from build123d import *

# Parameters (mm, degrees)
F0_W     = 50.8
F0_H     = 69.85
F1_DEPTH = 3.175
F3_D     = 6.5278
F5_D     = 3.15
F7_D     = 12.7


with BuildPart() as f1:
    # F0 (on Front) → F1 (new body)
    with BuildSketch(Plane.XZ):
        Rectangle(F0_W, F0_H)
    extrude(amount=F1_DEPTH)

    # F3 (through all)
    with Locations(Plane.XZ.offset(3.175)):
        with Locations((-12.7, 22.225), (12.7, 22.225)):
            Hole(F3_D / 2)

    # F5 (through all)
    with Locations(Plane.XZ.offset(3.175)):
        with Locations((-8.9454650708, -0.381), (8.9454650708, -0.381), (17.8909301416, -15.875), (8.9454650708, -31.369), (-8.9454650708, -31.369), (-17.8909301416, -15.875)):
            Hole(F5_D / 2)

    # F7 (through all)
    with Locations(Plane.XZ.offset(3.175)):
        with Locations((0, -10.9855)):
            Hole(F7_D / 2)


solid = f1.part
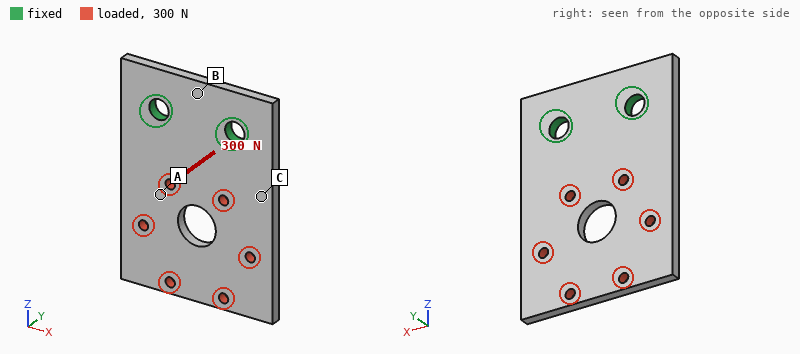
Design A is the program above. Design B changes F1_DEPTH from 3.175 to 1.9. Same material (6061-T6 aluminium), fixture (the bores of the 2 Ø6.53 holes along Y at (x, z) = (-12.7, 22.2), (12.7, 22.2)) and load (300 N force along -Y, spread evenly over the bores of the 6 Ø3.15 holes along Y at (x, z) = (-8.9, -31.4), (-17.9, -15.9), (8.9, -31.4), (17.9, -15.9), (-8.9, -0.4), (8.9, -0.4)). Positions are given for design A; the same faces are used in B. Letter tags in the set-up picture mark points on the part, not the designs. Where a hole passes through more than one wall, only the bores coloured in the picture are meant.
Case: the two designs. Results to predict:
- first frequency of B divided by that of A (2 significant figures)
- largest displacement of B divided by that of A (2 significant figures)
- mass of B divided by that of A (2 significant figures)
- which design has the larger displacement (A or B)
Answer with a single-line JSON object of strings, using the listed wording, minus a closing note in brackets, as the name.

{"first frequency of B divided by that of A": "0.61", "largest displacement of B divided by that of A": "4.5", "mass of B divided by that of A": "0.60", "which design has the larger displacement": "B"}
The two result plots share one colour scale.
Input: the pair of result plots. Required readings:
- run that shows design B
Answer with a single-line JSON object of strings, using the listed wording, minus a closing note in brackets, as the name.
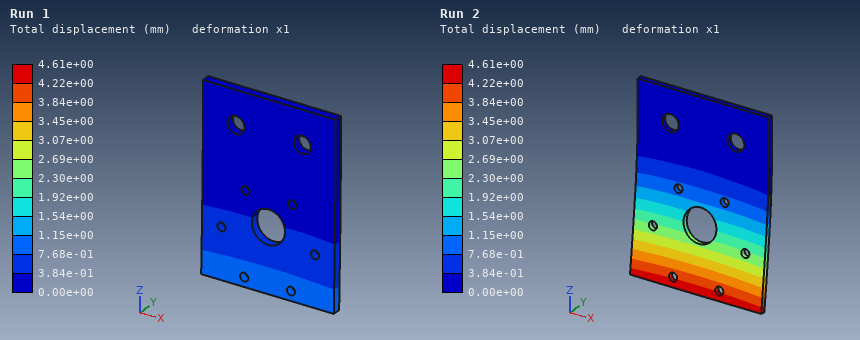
{"run that shows design B": "Run 2"}
